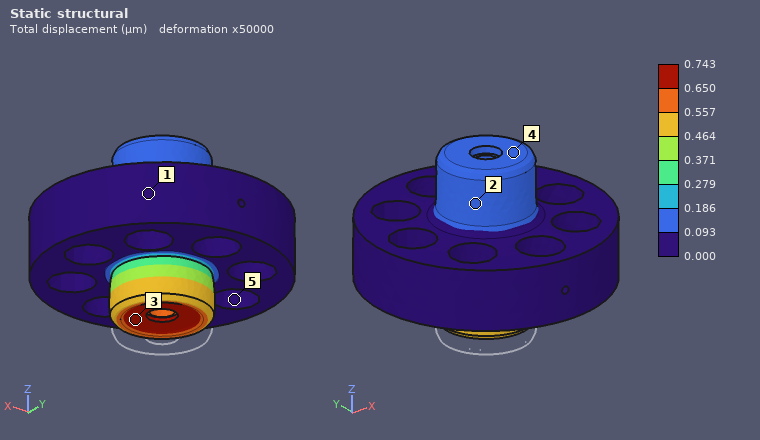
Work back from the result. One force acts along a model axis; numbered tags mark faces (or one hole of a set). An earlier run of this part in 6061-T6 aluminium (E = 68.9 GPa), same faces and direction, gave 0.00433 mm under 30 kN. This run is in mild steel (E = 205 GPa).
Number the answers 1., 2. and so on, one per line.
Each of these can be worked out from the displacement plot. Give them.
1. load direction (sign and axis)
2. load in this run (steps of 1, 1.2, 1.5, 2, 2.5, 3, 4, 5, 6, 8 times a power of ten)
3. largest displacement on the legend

1. +Z
2. 15 kN
3. 0.743 µm
